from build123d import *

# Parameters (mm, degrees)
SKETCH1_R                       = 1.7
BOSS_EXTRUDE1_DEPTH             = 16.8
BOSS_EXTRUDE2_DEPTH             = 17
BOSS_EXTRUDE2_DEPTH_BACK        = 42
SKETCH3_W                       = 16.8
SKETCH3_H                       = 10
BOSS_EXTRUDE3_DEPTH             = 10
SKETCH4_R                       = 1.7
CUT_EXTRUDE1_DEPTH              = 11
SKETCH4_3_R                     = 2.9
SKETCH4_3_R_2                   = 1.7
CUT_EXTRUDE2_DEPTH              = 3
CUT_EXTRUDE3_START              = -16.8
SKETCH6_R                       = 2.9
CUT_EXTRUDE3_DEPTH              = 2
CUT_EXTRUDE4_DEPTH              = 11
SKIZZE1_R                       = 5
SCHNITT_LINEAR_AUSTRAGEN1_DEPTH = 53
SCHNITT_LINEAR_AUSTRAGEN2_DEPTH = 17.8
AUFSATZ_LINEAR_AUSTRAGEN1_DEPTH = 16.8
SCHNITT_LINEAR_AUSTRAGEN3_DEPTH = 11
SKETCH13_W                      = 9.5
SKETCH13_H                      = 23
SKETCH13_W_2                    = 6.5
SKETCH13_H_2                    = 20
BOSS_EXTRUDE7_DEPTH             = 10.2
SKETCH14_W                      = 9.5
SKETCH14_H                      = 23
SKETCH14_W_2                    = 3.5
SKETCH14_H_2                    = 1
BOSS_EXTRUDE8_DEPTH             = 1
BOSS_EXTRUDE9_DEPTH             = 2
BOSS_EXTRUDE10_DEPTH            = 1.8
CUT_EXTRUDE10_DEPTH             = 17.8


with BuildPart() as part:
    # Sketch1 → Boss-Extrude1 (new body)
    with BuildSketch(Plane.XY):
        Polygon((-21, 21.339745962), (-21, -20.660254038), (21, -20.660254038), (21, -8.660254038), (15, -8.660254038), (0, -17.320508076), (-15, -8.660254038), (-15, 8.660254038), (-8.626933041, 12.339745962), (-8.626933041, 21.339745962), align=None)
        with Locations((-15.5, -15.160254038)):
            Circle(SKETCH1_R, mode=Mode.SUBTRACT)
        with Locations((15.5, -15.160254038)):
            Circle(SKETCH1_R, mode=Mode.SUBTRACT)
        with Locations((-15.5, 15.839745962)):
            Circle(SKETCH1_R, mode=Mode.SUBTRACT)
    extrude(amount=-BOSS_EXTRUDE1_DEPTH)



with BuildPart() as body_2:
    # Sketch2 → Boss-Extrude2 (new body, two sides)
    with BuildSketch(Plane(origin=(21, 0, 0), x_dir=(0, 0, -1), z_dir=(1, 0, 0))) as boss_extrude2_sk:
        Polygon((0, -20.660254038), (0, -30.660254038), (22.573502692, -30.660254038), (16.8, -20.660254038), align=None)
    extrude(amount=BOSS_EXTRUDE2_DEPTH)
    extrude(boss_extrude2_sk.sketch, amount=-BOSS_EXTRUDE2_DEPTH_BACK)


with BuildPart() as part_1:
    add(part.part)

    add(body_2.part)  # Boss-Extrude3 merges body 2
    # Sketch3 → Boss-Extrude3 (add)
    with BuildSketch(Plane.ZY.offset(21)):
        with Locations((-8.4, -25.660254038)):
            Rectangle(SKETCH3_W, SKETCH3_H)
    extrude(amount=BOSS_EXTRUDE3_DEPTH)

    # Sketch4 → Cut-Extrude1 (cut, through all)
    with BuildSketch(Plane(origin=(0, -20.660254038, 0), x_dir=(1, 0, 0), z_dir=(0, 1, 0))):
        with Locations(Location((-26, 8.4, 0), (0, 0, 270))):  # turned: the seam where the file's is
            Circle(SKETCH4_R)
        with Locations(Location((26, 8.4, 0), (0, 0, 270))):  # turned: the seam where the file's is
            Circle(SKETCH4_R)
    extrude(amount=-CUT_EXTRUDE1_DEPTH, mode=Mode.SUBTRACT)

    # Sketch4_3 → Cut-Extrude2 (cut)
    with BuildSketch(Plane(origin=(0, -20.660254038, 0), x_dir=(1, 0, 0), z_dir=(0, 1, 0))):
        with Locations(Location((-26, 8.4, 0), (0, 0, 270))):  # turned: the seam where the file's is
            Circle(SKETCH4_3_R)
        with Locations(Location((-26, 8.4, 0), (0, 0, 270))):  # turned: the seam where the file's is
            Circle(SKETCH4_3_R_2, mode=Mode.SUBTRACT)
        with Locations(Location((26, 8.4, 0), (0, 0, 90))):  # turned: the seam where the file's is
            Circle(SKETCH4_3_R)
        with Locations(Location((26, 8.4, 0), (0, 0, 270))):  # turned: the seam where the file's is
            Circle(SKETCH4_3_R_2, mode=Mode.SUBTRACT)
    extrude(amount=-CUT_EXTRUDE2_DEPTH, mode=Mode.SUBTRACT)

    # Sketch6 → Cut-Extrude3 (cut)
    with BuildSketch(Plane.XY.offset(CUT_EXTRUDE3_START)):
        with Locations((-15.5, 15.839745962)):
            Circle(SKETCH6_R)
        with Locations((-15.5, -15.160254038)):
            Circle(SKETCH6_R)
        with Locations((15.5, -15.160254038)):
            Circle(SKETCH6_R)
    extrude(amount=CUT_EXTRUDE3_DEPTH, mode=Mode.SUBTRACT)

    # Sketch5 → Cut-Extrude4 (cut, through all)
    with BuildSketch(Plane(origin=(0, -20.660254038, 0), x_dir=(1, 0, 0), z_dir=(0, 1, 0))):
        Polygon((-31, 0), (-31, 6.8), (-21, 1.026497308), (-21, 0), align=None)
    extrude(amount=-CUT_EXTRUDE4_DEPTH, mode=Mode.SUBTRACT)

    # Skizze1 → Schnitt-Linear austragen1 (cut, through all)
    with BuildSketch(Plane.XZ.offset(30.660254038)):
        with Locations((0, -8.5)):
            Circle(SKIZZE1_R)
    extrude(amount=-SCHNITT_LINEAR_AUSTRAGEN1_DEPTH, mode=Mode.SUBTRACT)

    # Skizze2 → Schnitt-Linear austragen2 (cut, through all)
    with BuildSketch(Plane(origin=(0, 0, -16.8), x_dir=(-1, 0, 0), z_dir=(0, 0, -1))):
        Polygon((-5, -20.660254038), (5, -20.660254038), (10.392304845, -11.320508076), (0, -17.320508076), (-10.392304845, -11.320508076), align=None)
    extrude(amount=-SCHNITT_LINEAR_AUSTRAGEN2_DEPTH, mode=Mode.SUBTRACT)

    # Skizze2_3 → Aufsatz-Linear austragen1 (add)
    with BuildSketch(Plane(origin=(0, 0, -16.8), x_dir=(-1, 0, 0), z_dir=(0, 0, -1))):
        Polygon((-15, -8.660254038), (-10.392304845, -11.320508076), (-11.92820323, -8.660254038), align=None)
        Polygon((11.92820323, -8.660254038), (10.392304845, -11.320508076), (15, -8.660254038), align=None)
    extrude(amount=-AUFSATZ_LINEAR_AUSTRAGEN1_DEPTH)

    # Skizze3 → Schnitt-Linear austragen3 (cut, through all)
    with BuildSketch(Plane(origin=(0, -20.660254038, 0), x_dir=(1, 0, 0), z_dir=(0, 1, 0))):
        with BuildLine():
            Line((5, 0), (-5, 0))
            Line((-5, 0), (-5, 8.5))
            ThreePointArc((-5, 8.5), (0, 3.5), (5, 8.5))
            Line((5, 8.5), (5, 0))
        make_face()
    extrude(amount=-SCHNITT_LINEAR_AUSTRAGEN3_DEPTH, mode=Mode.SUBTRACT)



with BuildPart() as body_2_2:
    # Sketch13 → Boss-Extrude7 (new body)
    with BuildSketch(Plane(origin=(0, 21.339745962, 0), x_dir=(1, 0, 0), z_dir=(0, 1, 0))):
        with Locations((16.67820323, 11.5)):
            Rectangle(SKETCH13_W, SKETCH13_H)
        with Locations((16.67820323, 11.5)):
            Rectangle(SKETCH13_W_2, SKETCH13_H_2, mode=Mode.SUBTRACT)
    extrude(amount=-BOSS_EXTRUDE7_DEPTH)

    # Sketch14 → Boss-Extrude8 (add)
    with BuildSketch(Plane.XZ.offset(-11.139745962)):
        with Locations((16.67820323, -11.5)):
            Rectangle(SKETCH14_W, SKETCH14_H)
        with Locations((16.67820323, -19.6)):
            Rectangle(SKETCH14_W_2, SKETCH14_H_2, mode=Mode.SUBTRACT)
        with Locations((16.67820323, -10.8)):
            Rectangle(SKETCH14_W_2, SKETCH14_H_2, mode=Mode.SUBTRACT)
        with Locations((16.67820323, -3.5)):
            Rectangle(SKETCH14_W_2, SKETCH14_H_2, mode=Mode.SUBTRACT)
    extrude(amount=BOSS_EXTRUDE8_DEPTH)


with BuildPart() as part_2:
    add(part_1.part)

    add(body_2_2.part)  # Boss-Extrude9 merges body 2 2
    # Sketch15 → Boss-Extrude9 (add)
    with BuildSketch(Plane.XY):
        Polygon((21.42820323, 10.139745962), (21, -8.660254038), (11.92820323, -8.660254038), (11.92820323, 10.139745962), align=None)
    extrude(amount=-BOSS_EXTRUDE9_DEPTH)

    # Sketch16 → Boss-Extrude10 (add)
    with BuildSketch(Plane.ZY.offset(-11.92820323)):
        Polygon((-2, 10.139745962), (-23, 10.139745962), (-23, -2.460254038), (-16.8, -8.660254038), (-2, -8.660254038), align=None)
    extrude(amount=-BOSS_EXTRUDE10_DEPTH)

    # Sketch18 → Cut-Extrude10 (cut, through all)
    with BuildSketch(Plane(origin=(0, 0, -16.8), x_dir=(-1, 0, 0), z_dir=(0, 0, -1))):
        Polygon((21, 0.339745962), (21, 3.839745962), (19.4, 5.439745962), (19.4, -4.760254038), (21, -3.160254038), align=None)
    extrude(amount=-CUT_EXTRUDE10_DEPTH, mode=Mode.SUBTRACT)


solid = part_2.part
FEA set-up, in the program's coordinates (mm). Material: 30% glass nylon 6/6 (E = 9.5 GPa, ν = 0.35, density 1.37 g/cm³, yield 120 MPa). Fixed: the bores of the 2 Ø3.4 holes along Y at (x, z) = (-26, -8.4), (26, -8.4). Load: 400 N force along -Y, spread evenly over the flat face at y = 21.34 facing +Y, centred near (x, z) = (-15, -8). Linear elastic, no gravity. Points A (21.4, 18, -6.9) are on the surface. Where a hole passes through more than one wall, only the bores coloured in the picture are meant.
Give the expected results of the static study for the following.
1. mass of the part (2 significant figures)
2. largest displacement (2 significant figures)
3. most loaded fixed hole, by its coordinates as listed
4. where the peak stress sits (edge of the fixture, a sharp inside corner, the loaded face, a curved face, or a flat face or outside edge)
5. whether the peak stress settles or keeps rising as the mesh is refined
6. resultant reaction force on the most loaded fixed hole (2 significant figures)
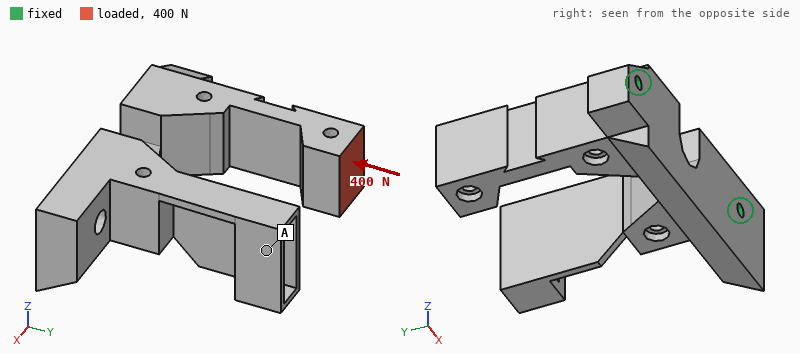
30 g
0.43 mm
(-26, -8.4)
edge of the fixture
keeps rising
330 N
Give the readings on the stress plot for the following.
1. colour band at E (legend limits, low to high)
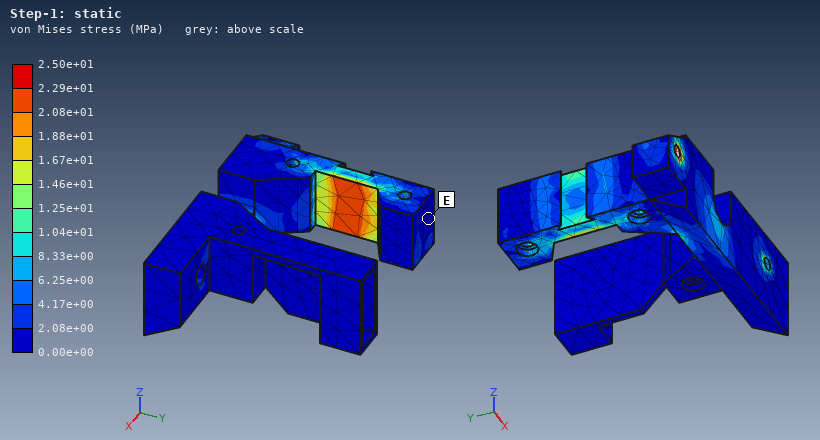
0.00e+00 to 2.08e+00 MPa
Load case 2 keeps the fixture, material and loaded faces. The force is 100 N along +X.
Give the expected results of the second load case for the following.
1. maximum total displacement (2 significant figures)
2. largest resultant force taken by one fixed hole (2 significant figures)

0.91 mm
110 N
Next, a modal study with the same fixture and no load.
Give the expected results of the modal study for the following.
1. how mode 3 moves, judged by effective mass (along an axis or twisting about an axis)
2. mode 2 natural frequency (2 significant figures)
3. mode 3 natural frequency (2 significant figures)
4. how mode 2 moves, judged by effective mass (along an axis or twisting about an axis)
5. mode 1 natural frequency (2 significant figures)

along Z
1200 Hz
1500 Hz
along X
1100 Hz
